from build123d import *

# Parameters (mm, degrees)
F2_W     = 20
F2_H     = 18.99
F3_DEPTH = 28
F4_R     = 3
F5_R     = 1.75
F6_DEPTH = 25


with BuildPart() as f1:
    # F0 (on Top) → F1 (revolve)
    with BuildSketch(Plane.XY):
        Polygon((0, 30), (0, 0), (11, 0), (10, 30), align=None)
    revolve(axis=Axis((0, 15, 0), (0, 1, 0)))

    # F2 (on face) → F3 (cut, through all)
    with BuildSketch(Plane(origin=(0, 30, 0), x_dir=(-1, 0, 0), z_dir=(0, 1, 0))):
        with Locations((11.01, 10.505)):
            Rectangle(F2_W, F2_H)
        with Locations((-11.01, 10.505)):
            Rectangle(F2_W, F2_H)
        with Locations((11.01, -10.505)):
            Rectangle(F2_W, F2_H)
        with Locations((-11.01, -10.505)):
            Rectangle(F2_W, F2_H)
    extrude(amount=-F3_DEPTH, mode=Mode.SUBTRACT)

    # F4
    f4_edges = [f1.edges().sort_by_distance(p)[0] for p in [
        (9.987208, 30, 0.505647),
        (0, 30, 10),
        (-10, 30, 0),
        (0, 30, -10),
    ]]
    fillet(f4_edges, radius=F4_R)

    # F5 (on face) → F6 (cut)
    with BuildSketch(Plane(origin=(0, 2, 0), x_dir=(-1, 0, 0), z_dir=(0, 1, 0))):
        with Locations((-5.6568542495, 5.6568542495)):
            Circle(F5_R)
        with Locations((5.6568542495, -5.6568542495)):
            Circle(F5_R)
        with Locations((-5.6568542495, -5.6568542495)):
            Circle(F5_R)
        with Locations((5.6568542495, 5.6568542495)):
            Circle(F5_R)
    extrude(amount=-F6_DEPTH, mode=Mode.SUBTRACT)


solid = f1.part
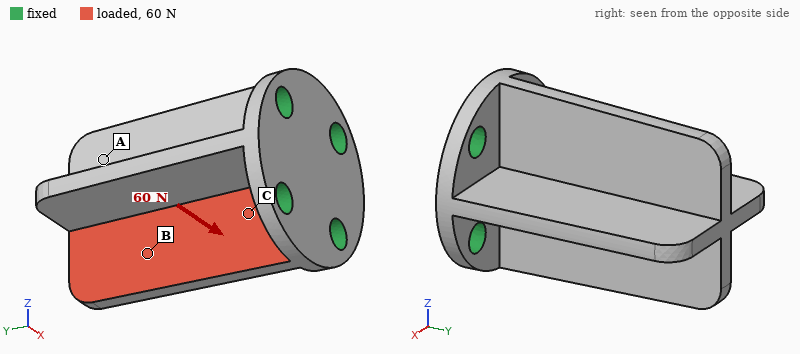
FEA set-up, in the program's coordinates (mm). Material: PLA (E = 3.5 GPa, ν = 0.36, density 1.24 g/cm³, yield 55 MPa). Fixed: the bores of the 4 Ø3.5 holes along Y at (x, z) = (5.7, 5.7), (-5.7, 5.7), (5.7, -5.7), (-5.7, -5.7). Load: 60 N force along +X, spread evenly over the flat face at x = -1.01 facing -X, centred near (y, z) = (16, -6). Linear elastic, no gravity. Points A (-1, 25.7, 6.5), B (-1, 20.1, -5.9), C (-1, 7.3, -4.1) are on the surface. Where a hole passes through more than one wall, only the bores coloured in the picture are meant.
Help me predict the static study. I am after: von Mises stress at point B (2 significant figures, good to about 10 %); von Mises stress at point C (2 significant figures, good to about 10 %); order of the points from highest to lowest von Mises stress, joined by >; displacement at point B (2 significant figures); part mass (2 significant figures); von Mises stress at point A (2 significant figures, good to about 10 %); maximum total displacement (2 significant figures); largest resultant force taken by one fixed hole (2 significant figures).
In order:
4.6 MPa
7.4 MPa
C > B > A
0.21 mm
3.6 g
2.2 MPa
0.40 mm
44 N
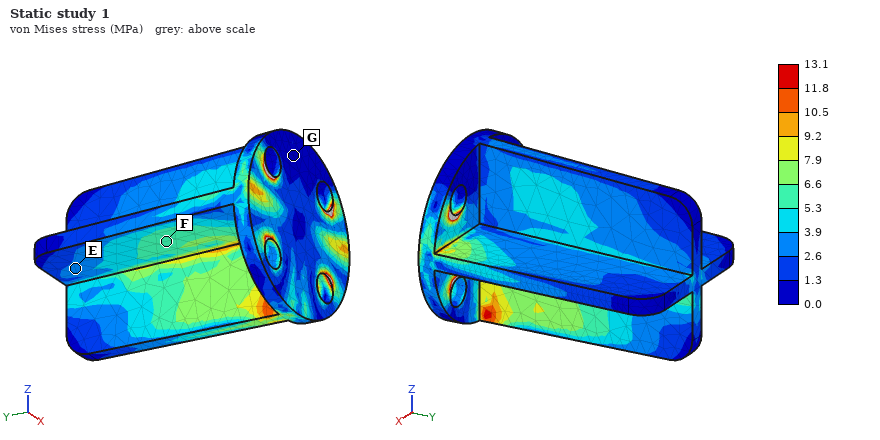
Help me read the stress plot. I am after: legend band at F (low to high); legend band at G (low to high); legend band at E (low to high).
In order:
5.3 to 6.6 MPa
0.0 to 1.3 MPa
2.6 to 3.9 MPa
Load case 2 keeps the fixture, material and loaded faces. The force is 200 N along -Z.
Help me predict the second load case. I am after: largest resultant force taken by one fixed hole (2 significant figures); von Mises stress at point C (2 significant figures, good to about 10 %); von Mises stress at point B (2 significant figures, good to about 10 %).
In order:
130 N
15 MPa
7.9 MPa
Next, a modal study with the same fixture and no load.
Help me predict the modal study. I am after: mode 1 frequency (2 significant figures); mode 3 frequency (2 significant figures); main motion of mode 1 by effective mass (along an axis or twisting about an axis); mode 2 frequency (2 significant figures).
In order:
2200 Hz
2500 Hz
twisting about Y
2500 Hz
